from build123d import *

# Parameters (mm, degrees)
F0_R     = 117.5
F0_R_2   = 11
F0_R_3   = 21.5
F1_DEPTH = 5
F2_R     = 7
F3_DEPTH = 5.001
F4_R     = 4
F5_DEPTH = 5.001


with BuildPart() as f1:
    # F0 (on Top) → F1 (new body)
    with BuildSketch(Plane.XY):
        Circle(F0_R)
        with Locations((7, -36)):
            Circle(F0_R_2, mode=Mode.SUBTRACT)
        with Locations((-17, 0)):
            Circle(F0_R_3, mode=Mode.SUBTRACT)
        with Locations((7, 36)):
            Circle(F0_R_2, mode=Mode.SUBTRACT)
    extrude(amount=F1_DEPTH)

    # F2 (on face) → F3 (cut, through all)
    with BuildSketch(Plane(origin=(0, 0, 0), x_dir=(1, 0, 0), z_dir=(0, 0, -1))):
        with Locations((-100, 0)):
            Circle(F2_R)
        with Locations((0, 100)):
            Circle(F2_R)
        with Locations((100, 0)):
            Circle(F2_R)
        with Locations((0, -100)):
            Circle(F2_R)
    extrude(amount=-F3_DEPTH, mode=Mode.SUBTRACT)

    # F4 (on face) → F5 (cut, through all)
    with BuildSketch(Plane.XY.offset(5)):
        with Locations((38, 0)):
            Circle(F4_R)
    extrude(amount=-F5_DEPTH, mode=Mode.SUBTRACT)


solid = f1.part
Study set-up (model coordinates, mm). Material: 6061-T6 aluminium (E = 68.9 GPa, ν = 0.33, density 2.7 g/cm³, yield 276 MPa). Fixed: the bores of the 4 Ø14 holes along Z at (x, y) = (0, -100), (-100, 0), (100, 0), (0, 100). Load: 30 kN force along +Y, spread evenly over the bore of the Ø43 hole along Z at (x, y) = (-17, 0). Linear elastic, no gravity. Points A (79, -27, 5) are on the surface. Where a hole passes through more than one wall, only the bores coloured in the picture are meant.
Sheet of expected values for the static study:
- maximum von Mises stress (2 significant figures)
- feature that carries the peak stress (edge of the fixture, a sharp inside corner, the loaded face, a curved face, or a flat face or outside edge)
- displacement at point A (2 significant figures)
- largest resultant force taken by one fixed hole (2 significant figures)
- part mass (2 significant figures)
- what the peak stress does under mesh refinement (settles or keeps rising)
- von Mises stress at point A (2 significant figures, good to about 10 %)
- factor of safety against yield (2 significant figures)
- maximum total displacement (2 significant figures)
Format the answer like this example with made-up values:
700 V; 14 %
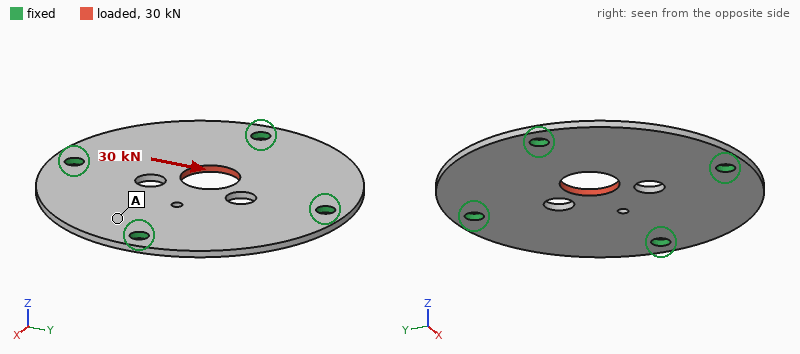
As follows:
140 MPa; a curved face; 13 µm; 9.2 kN; 550 g; settles; 9.8 MPa; 2.0; 70 µm
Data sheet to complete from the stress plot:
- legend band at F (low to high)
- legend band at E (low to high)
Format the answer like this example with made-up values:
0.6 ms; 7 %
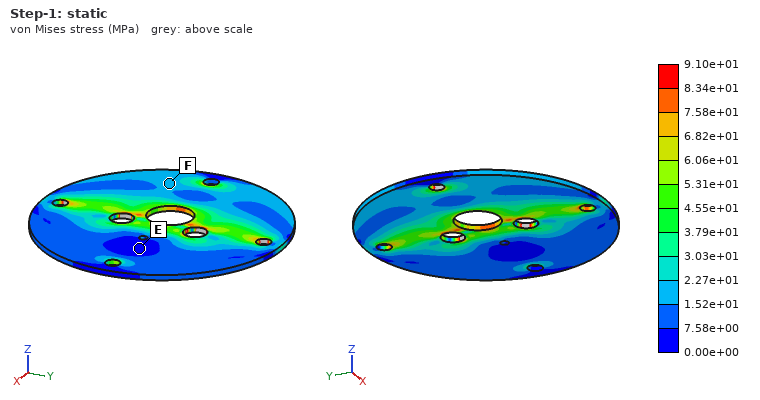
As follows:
1.52e+01 to 2.27e+01 MPa; 0.00e+00 to 7.58e+00 MPa
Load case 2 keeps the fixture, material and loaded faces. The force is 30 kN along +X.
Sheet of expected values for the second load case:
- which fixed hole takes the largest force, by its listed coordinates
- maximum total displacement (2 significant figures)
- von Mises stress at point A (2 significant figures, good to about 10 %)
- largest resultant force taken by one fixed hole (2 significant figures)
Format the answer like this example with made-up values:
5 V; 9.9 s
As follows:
(-100, 0); 60 µm; 18 MPa; 12 kN
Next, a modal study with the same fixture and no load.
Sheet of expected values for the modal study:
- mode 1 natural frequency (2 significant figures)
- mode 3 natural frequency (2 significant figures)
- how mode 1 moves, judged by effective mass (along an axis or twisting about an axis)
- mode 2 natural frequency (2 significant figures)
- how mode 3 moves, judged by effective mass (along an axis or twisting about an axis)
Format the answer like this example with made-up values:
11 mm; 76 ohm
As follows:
1000 Hz; 1200 Hz; along Z; 1100 Hz; twisting about X
